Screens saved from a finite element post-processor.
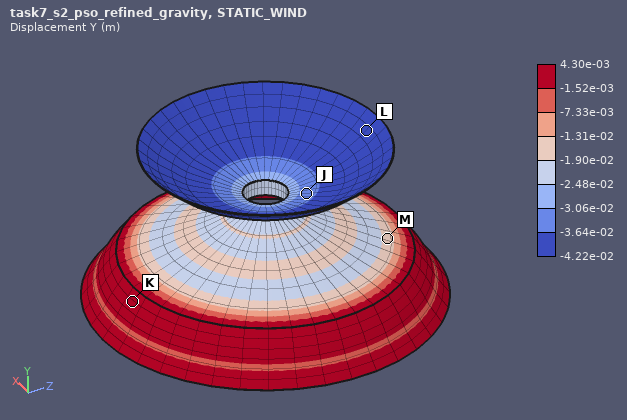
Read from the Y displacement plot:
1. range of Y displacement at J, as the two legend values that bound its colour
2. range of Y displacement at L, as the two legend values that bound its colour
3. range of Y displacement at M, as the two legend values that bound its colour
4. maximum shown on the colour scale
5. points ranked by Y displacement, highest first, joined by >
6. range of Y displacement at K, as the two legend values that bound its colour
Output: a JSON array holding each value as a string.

["-3.64e-02 to -3.06e-02 m", "-4.22e-02 to -3.64e-02 m", "-1.90e-02 to -1.31e-02 m", "4.30e-03 m", "K > M > J > L", "-1.52e-03 to 4.30e-03 m"]
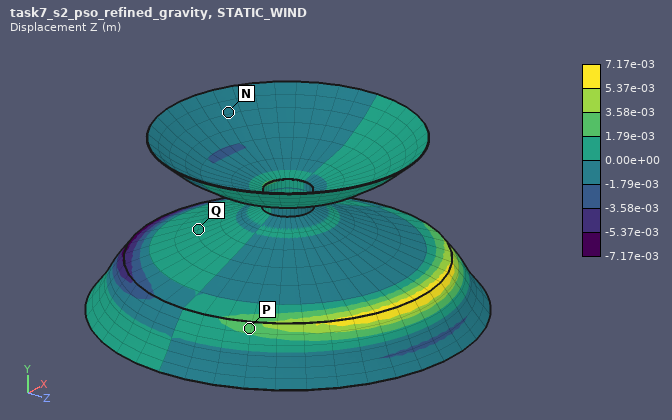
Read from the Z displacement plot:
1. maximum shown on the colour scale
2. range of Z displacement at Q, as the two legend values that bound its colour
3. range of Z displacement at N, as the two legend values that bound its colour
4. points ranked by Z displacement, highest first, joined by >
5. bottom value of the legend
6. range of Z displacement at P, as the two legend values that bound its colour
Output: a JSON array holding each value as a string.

["7.17e-03 m", "0.00e+00 to 1.79e-03 m", "-1.79e-03 to 0.00e+00 m", "P > Q > N", "-7.17e-03 m", "1.79e-03 to 3.58e-03 m"]
